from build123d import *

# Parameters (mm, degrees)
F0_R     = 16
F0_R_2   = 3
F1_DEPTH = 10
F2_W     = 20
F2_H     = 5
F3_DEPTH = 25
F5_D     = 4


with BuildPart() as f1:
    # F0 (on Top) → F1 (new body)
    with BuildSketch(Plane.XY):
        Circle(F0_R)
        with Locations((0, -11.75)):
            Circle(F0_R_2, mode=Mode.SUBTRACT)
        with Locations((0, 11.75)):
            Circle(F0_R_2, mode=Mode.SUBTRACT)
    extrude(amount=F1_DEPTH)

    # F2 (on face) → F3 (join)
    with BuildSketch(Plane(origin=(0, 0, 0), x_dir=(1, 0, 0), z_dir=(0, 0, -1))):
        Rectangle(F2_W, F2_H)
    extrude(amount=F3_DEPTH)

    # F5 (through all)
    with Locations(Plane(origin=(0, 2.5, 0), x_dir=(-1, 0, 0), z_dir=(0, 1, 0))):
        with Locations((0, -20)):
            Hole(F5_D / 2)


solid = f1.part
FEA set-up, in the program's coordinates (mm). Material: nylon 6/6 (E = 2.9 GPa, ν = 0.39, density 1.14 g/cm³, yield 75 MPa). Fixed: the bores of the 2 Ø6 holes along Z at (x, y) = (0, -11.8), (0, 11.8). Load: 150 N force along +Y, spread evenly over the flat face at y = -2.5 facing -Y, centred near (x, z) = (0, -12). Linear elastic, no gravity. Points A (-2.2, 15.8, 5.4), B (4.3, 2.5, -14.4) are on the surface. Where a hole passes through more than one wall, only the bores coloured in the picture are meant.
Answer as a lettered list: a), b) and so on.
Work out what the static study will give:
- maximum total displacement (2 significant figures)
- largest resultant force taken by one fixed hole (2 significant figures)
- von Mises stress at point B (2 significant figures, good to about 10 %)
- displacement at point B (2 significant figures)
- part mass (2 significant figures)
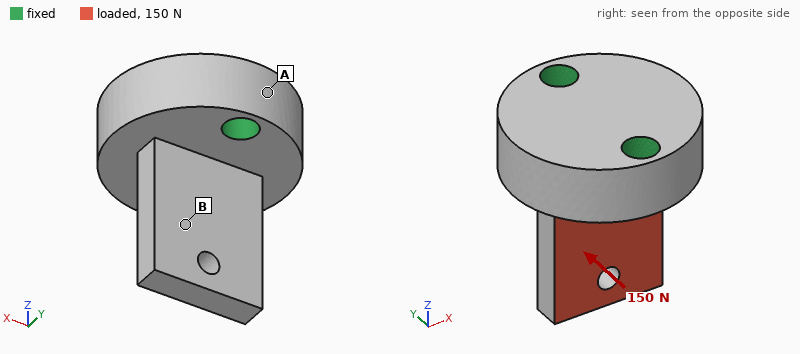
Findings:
a) 0.59 mm
b) 150 N
c) 4.1 MPa
d) 0.29 mm
e) 11 g
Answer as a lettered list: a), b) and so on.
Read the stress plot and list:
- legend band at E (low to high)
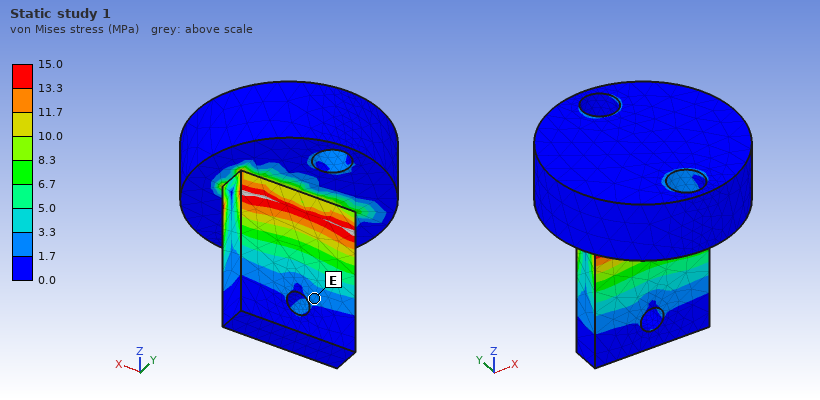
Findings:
a) 1.7 to 3.3 MPa
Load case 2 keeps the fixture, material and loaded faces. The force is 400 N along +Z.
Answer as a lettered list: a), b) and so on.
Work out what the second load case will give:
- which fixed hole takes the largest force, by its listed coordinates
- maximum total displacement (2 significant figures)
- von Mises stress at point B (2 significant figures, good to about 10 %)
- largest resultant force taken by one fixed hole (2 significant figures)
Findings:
a) (0, -11.8)
b) 0.40 mm
c) 3.2 MPa
d) 250 N
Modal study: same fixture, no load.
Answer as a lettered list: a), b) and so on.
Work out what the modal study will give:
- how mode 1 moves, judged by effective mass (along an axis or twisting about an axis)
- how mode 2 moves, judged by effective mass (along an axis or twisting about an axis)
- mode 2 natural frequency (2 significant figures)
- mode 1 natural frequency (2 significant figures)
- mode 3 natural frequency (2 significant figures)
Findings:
a) along Y
b) along X
c) 3900 Hz
d) 1900 Hz
e) 4700 Hz
